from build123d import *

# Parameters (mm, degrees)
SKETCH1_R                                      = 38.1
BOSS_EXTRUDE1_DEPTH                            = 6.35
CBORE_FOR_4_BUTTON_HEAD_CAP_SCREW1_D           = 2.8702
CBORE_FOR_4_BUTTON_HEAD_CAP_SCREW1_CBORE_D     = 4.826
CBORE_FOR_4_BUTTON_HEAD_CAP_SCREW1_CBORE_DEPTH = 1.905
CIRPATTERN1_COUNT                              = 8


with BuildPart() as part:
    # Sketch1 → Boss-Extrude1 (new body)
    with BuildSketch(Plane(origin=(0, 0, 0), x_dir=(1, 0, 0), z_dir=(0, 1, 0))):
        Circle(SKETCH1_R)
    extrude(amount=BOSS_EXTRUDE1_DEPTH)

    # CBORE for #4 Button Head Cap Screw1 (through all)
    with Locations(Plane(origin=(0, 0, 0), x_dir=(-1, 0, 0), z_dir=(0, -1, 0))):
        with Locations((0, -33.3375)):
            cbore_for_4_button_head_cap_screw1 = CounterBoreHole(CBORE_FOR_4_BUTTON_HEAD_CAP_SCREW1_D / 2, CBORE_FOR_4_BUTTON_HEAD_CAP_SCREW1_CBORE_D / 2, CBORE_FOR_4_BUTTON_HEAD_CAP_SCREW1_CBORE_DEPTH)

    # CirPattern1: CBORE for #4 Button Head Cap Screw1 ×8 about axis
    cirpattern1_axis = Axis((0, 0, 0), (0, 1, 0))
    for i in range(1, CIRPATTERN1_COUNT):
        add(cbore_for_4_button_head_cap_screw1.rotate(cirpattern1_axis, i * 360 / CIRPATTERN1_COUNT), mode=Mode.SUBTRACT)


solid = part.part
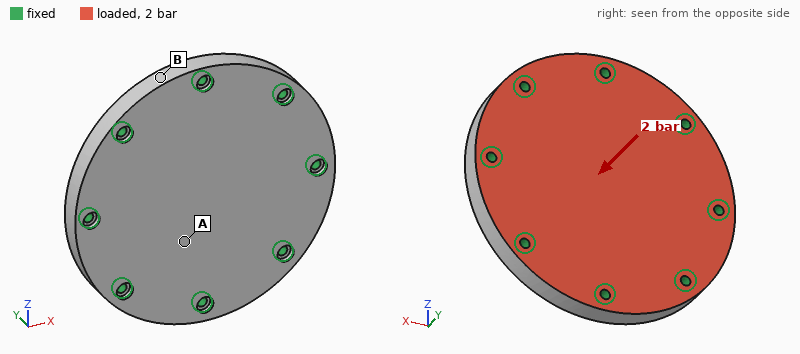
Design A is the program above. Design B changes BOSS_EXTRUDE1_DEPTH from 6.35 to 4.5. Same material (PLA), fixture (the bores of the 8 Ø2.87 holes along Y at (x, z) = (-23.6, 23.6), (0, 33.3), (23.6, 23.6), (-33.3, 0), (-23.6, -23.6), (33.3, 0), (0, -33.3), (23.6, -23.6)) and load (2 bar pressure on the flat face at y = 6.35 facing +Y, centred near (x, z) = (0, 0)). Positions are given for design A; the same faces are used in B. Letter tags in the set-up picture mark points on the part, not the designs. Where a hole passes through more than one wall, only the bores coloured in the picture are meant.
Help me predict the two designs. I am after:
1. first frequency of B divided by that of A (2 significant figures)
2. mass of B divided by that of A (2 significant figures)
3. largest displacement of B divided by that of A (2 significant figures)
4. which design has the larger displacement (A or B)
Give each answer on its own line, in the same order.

0.74
0.71
2.6
B
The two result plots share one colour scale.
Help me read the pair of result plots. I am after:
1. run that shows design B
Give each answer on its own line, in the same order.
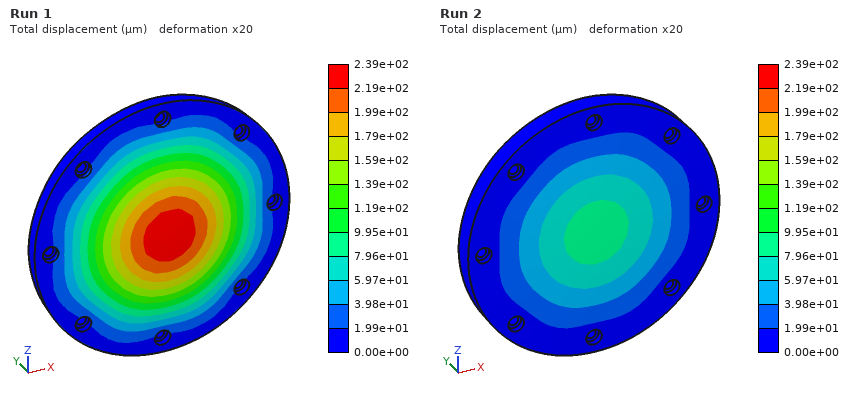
Run 1
